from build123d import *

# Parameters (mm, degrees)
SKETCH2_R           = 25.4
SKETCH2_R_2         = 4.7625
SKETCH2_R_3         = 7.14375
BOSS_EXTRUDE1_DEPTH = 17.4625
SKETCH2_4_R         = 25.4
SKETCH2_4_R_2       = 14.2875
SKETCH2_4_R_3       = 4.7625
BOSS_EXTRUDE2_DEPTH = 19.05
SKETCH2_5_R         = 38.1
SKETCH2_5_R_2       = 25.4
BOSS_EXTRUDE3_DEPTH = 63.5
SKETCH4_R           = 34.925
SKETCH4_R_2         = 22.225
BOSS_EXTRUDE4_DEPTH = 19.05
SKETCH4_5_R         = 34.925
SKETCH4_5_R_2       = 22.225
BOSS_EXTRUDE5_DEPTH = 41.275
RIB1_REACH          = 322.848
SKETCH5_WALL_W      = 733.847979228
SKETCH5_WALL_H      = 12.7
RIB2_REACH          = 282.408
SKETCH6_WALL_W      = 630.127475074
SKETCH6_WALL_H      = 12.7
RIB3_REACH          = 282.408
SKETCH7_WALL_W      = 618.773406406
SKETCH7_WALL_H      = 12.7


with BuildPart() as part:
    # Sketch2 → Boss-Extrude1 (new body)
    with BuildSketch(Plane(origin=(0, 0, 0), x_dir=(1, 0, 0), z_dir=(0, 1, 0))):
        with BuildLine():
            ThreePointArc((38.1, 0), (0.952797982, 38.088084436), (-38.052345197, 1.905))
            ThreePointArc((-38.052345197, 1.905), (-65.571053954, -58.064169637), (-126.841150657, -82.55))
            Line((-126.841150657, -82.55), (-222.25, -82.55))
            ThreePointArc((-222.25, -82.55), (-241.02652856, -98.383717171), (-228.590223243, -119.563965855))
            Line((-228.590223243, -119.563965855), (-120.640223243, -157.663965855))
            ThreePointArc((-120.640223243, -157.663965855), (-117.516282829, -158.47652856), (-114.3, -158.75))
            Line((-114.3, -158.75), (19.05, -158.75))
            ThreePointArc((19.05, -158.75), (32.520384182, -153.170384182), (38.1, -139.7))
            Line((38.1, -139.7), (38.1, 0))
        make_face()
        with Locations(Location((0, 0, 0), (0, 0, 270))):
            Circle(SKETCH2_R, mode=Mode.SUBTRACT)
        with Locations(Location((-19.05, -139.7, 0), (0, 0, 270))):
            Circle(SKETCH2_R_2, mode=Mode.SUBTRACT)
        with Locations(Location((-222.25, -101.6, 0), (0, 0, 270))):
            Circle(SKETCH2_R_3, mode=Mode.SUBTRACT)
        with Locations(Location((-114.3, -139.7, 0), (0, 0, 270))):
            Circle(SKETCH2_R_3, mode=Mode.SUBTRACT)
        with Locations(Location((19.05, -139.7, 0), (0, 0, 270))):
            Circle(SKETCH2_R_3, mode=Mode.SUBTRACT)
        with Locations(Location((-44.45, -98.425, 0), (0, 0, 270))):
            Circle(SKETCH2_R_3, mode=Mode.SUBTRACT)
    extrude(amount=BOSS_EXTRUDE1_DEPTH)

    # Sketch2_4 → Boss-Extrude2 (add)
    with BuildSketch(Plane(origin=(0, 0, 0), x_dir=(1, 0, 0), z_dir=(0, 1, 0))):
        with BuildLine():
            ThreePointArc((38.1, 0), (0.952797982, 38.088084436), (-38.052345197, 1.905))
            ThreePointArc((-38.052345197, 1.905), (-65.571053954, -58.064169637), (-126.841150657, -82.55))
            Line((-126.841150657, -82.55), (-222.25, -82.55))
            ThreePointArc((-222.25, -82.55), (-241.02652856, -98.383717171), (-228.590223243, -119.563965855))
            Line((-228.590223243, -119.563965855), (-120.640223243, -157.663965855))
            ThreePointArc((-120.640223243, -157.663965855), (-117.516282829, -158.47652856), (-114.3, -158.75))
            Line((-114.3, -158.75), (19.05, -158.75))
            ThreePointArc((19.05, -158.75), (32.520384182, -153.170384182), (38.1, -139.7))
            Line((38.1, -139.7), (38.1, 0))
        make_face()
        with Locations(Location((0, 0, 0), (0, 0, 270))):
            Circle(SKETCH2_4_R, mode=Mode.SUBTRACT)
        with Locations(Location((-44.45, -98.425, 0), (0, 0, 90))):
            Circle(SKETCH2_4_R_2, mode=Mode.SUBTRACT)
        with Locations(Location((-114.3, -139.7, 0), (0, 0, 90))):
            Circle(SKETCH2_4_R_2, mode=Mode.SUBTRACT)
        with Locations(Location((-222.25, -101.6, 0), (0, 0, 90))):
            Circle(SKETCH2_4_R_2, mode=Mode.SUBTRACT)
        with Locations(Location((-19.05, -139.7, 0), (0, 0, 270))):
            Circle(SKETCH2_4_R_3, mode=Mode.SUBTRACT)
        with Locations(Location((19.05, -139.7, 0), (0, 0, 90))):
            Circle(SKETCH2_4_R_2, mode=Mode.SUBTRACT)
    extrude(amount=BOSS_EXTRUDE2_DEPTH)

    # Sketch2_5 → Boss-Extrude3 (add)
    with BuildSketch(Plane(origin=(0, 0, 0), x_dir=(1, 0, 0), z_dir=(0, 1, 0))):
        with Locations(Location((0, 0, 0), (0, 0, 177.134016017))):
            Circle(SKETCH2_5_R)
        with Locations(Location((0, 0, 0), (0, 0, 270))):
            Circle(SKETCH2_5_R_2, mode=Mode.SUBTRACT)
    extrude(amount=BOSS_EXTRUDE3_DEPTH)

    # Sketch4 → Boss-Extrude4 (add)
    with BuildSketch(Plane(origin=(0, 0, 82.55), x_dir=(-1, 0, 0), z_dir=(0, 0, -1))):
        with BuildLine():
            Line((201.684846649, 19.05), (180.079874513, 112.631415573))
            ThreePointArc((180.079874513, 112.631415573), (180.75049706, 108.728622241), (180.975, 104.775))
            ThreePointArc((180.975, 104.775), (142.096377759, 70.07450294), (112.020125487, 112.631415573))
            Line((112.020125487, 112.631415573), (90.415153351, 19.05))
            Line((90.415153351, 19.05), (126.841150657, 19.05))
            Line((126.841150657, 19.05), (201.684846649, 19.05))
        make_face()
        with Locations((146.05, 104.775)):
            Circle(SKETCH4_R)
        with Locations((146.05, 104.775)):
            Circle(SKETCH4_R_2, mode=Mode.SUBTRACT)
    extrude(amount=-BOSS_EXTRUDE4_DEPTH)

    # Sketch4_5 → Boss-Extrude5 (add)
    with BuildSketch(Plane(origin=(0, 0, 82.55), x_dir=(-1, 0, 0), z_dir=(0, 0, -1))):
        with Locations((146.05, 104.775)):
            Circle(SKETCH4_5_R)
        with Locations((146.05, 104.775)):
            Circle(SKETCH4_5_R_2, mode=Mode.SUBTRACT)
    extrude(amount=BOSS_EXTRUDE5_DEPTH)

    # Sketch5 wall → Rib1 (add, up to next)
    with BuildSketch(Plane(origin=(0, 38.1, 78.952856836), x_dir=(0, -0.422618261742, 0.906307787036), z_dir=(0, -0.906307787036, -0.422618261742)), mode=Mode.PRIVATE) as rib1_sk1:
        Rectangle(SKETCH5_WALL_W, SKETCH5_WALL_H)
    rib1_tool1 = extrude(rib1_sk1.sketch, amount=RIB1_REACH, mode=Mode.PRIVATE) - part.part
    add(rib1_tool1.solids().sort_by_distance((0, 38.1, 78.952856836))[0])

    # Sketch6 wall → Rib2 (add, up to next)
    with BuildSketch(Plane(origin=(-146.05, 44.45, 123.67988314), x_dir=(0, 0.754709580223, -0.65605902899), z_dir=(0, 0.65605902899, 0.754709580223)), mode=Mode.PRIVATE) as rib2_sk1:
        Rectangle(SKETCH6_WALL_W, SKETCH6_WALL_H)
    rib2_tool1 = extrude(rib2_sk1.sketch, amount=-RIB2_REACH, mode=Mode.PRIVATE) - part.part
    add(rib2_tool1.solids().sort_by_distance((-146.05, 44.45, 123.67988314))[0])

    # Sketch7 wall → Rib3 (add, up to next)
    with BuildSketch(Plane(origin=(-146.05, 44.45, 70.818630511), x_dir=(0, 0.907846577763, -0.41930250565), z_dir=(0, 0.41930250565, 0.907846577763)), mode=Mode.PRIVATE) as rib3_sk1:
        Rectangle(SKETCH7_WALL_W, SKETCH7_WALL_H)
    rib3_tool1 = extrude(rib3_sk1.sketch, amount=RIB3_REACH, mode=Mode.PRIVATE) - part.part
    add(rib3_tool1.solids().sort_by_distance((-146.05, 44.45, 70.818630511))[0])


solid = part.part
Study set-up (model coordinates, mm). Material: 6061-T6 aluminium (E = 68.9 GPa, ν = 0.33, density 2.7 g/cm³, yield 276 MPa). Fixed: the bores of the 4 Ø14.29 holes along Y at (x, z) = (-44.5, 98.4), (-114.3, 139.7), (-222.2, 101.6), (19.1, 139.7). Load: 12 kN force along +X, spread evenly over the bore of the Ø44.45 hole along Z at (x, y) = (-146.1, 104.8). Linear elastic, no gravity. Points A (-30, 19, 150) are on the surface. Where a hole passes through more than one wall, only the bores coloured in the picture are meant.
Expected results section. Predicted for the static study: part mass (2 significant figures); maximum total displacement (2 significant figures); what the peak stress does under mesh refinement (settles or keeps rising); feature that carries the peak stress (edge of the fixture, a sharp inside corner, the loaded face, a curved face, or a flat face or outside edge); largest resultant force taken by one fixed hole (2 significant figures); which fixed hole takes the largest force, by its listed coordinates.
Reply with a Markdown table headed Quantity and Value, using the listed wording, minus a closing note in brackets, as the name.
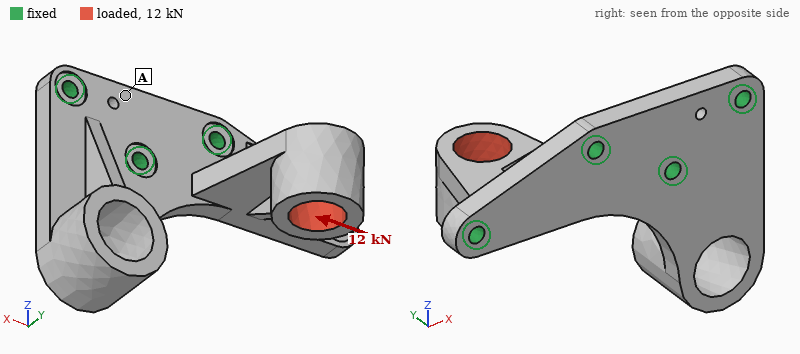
| Quantity | Value |
|---|---|
| part mass | 2.4 kg |
| maximum total displacement | 0.25 mm |
| what the peak stress does under mesh refinement | keeps rising |
| feature that carries the peak stress | edge of the fixture |
| largest resultant force taken by one fixed hole | 11 kN |
| which fixed hole takes the largest force, by its listed coordinates | (-222.2, 101.6) |
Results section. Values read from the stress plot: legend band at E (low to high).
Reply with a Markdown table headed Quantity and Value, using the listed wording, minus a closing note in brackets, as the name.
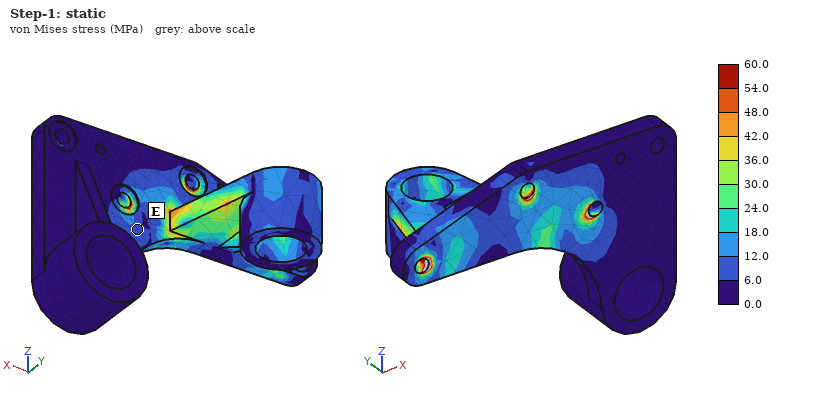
| Quantity | Value |
|---|---|
| legend band at E | 6.0 to 12.0 MPa |
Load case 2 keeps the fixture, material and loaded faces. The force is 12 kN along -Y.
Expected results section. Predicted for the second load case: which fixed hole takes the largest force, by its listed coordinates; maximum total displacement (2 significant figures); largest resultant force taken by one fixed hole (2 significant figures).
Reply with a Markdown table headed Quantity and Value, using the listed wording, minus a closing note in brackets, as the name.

| Quantity | Value |
|---|---|
| which fixed hole takes the largest force, by its listed coordinates | (-222.2, 101.6) |
| maximum total displacement | 0.45 mm |
| largest resultant force taken by one fixed hole | 7.9 kN |
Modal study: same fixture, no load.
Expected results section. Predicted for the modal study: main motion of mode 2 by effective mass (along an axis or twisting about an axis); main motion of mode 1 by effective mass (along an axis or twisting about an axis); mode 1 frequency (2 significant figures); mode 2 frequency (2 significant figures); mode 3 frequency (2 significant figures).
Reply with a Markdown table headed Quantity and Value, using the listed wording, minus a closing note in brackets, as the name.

| Quantity | Value |
|---|---|
| main motion of mode 2 by effective mass | along Z |
| main motion of mode 1 by effective mass | along Y |
| mode 1 frequency | 720 Hz |
| mode 2 frequency | 940 Hz |
| mode 3 frequency | 1800 Hz |
